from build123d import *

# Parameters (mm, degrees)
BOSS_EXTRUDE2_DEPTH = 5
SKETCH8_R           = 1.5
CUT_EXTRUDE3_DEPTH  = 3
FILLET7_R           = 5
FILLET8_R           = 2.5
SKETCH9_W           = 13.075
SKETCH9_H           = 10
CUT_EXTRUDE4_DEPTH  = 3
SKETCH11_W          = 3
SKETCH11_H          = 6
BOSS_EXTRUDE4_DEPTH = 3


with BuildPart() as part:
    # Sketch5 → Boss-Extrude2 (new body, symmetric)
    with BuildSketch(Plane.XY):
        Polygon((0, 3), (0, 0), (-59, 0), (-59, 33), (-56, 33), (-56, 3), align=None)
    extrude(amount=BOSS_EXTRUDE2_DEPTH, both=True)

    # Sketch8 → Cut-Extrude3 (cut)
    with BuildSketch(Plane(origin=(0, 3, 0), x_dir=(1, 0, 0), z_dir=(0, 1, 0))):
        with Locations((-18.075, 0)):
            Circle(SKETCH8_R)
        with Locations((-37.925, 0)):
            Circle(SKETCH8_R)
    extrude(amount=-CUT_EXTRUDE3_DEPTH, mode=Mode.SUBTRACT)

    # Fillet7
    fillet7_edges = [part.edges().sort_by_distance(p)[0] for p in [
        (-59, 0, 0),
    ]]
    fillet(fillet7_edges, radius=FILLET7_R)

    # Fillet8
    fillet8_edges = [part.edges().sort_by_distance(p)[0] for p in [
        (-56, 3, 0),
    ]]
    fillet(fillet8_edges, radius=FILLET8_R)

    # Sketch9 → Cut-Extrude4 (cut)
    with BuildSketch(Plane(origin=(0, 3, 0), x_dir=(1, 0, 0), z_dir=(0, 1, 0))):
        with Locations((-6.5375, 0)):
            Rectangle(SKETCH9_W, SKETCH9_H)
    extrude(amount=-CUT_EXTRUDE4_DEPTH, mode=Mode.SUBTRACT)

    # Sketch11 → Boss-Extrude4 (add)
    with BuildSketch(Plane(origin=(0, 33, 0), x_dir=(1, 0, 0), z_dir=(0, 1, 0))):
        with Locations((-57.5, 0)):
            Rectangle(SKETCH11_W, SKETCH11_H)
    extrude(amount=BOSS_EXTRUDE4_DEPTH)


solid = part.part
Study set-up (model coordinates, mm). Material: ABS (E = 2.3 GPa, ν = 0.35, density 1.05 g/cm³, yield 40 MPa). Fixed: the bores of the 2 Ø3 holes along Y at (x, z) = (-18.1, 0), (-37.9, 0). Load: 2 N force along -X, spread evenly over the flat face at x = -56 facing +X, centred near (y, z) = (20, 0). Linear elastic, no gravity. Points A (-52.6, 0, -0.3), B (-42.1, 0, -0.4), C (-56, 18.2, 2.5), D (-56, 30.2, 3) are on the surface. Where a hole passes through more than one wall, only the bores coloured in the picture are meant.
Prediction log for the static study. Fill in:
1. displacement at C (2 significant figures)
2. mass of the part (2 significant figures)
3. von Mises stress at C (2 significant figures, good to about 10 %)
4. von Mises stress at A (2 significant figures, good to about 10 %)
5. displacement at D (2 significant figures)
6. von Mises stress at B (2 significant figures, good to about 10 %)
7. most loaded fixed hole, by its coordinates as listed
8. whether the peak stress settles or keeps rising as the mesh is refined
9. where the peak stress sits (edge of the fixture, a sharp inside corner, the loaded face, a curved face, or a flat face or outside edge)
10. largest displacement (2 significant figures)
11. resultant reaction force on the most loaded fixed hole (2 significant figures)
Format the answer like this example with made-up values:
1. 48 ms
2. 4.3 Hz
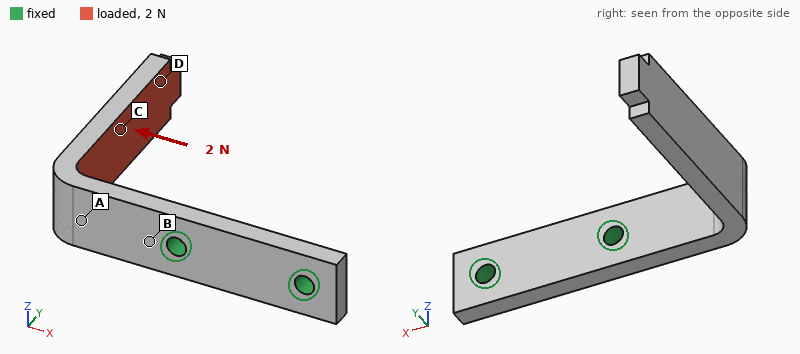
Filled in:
1. 0.29 mm
2. 2.4 g
3. 0.64 MPa
4. 2.2 MPa
5. 0.51 mm
6. 2.5 MPa
7. (-37.9, 0)
8. keeps rising
9. edge of the fixture
10. 0.64 mm
11. 1.9 N
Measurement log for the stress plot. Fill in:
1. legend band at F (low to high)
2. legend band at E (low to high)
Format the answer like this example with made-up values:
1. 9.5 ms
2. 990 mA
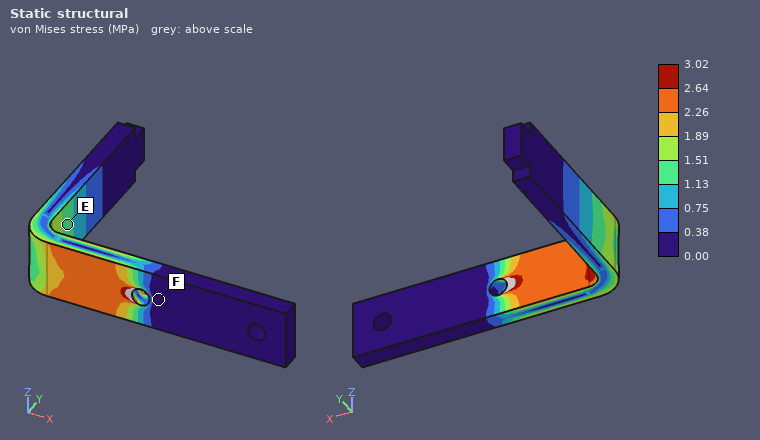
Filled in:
1. 0.00 to 0.38 MPa
2. 1.13 to 1.51 MPa
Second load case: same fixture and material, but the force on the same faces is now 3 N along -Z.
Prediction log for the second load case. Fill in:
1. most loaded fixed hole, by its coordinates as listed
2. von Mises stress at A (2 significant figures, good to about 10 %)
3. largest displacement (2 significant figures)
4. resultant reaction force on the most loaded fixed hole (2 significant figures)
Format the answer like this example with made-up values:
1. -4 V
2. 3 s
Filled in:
1. (-37.9, 0)
2. 3.2 MPa
3. 0.56 mm
4. 4.4 N
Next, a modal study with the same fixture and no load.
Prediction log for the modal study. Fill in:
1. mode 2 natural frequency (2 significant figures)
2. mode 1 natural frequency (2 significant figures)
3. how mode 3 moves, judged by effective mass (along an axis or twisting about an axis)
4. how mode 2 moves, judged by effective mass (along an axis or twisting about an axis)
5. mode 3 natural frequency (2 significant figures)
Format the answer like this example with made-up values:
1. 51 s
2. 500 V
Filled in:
1. 470 Hz
2. 340 Hz
3. along Y
4. along Z
5. 1100 Hz
